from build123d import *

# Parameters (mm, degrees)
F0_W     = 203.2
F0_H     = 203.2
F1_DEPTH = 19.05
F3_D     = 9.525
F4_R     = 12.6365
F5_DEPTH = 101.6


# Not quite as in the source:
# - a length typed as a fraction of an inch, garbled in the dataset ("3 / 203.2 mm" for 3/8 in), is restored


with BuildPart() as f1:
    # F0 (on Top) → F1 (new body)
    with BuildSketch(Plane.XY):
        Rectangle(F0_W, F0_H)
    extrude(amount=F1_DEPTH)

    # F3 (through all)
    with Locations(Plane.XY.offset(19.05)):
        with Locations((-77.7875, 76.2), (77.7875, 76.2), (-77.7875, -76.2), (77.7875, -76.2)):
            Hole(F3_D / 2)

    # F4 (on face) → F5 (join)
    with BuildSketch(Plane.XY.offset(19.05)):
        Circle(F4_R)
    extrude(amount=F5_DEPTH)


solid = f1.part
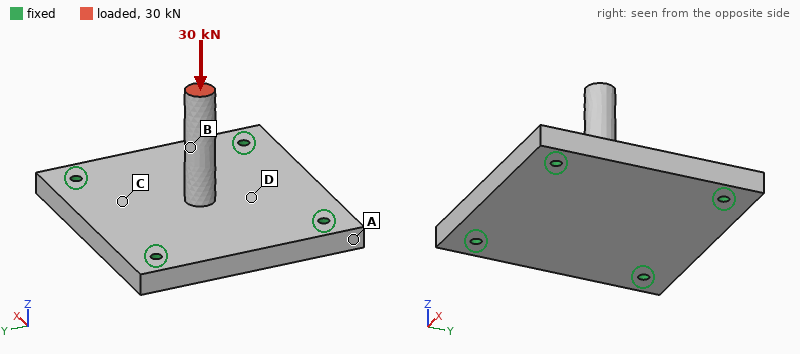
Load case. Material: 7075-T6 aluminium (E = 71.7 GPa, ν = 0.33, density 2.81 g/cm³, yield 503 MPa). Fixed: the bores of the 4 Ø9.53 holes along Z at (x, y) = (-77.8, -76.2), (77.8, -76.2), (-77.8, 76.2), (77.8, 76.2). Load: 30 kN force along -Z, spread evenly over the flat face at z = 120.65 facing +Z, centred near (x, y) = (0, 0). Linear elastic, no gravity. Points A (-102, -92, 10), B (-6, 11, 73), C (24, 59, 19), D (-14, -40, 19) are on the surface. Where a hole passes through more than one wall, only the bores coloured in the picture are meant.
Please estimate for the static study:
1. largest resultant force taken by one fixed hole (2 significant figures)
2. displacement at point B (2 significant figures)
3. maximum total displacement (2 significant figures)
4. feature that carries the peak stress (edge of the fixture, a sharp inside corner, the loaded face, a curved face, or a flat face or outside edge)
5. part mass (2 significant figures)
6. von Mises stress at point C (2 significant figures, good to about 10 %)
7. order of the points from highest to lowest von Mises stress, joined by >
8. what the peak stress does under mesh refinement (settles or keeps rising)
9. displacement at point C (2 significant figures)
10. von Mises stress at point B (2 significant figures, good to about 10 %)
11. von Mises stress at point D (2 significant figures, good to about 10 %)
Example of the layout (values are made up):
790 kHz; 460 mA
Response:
7.5 kN; 0.28 mm; 0.32 mm; edge of the fixture; 2.3 kg; 28 MPa; B > D > C > A; keeps rising; 0.11 mm; 60 MPa; 42 MPa
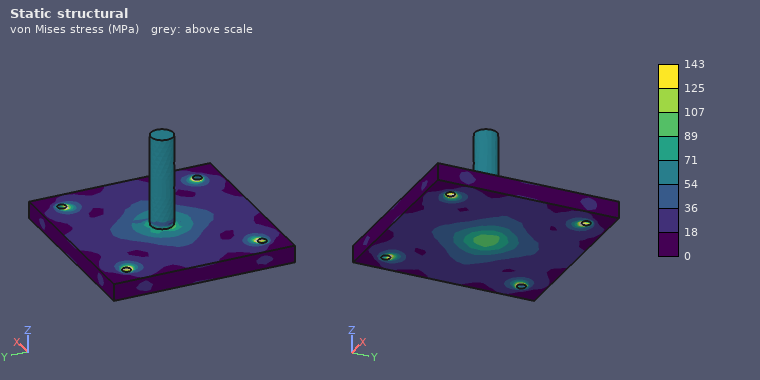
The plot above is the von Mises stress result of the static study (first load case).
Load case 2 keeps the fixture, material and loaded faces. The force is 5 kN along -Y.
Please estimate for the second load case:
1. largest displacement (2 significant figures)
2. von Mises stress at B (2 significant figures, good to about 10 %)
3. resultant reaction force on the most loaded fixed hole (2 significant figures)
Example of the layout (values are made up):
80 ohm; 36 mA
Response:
1.7 mm; 140 MPa; 2.5 kN
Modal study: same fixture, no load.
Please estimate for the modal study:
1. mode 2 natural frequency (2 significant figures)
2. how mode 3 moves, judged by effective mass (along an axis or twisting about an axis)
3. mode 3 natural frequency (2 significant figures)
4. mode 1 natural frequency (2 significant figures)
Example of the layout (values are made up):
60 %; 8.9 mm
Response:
1400 Hz; along Z; 2200 Hz; 1400 Hz
